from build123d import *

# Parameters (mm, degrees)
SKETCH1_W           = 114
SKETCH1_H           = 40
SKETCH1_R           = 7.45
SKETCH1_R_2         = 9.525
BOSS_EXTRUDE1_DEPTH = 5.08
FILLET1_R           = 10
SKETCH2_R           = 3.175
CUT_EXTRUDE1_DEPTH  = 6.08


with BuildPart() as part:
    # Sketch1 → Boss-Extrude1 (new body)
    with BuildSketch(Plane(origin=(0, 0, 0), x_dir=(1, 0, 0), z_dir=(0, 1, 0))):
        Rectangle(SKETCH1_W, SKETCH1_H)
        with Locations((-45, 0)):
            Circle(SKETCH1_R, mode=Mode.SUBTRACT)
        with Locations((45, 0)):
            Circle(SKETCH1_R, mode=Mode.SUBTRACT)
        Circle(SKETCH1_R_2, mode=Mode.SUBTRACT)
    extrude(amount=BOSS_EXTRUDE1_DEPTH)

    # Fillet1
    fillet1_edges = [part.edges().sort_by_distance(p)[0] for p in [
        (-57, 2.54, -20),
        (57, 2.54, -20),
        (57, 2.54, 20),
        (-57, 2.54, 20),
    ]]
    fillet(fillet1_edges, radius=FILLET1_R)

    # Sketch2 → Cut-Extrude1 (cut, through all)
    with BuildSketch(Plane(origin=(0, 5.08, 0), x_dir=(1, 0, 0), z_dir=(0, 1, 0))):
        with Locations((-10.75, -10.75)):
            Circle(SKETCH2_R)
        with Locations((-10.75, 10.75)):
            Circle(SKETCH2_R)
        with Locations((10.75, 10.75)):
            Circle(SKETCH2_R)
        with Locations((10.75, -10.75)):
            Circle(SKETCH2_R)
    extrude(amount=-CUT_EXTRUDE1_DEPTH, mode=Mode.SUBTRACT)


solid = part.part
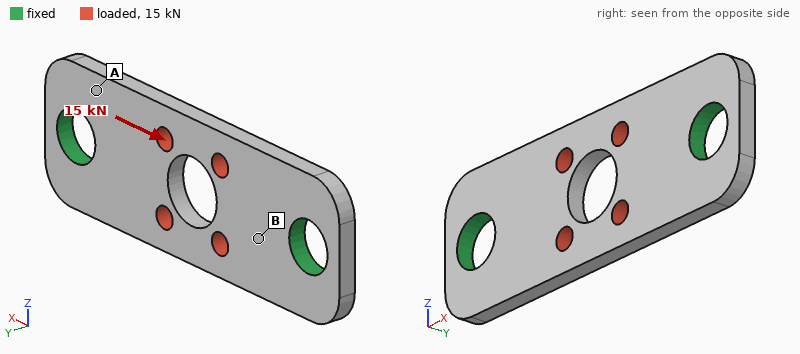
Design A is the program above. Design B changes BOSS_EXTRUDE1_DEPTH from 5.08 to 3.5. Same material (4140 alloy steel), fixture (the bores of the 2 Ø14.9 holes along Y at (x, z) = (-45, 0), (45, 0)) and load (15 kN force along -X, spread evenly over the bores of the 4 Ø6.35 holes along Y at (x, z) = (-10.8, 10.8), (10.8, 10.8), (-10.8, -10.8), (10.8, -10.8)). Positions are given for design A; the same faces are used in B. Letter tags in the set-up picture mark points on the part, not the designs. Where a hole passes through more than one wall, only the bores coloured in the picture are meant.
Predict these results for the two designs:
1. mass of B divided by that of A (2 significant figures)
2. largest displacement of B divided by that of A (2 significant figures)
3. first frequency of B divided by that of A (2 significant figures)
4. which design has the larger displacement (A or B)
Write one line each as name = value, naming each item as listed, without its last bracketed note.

mass of B divided by that of A = 0.69
largest displacement of B divided by that of A = 1.5
first frequency of B divided by that of A = 0.71
which design has the larger displacement = B
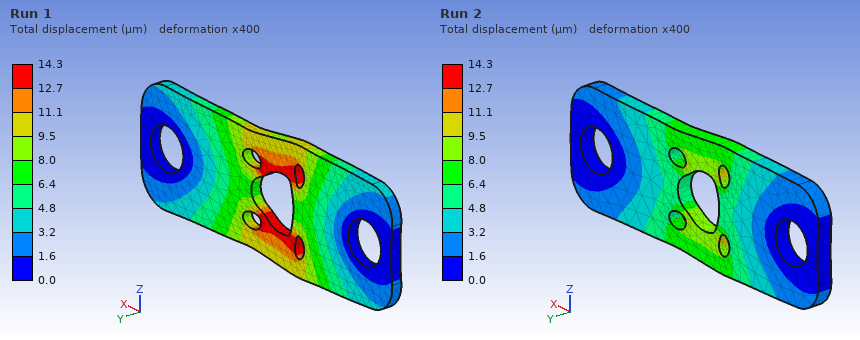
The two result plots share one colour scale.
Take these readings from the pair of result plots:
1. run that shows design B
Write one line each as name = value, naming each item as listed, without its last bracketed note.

run that shows design B = Run 1
